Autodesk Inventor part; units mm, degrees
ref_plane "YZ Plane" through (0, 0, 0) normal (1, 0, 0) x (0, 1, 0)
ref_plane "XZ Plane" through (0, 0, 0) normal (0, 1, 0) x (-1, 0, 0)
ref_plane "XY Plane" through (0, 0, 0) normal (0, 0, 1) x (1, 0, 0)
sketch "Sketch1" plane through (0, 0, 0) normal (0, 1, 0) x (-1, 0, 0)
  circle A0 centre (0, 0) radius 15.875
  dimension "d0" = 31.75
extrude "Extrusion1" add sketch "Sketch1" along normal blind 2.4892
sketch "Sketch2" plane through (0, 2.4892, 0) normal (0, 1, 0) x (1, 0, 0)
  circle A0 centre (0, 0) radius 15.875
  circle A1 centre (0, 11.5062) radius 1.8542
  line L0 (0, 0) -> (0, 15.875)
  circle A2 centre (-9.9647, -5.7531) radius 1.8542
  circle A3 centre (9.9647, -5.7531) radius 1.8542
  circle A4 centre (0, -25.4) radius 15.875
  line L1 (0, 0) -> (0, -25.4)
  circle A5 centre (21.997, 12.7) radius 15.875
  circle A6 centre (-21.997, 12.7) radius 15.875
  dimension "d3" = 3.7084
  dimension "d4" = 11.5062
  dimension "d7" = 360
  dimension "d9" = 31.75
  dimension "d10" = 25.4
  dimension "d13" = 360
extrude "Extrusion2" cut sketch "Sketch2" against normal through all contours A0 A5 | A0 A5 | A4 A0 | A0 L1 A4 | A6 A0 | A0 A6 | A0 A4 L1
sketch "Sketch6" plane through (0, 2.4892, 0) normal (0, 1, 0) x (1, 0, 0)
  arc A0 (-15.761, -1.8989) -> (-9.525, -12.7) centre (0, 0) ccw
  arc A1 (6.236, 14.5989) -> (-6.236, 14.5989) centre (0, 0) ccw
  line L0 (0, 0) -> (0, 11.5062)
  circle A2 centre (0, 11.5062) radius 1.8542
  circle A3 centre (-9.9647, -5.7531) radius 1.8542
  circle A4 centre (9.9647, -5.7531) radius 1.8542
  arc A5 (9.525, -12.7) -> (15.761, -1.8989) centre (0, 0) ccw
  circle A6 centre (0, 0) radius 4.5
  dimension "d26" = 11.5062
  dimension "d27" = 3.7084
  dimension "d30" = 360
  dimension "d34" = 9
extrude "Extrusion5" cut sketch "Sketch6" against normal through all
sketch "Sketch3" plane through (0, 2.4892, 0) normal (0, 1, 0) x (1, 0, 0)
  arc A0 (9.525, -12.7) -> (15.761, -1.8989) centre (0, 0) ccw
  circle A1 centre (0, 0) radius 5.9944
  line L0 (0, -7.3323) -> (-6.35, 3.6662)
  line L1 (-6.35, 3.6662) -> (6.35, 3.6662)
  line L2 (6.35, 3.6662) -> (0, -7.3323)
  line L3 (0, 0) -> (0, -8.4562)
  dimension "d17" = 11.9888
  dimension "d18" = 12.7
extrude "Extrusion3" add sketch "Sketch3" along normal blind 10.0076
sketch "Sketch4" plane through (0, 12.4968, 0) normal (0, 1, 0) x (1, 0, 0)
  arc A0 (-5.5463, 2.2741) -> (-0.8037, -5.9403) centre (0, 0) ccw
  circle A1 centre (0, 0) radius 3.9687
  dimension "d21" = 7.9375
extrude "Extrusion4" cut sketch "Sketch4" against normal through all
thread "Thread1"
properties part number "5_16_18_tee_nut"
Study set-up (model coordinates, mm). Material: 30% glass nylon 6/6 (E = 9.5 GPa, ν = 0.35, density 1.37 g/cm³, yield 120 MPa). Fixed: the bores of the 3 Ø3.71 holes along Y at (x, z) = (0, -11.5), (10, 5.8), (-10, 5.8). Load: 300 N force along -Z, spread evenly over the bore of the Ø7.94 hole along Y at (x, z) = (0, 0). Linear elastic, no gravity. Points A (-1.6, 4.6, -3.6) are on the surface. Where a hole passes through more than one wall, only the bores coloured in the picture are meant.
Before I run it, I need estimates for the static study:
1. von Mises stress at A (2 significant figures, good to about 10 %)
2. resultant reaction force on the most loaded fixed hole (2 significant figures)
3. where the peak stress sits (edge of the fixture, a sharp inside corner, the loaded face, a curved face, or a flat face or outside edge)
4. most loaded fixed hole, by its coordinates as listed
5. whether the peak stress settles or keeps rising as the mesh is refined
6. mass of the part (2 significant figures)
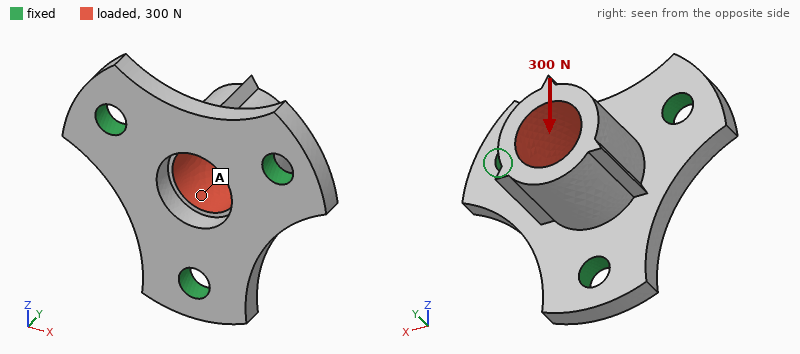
9.1 MPa
180 N
edge of the fixture
(0, -11.5)
keeps rising
2.4 g
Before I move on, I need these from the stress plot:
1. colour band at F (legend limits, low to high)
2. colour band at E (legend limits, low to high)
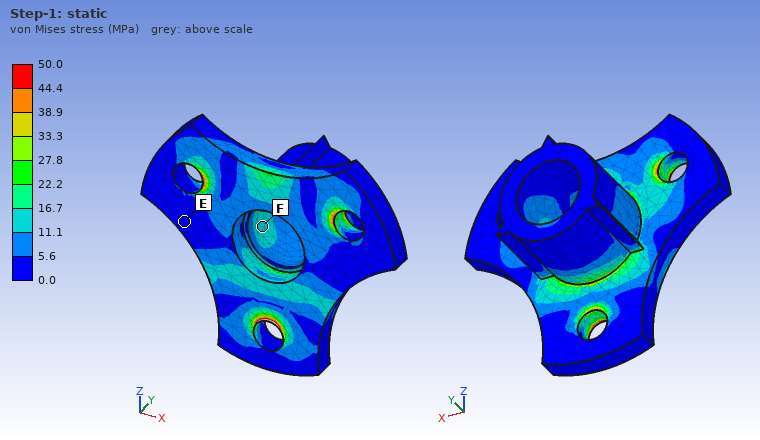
11.1 to 16.7 MPa
0.0 to 5.6 MPa
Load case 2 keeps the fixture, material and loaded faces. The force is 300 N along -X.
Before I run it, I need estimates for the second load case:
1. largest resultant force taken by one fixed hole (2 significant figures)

160 N
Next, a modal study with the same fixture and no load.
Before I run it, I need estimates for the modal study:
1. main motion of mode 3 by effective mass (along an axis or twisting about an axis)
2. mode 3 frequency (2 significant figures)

along Y
15 kHz
